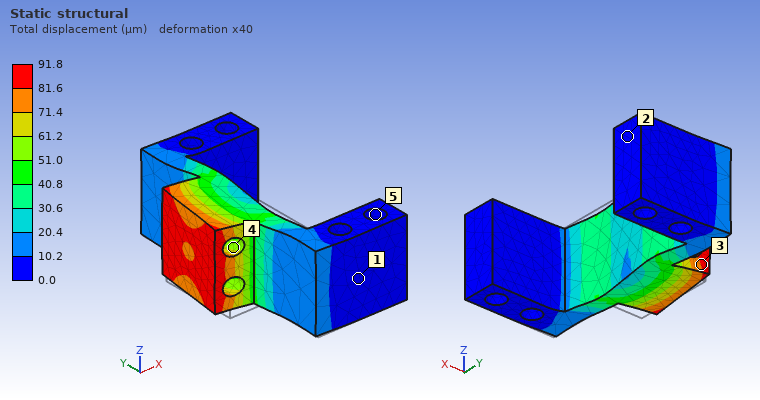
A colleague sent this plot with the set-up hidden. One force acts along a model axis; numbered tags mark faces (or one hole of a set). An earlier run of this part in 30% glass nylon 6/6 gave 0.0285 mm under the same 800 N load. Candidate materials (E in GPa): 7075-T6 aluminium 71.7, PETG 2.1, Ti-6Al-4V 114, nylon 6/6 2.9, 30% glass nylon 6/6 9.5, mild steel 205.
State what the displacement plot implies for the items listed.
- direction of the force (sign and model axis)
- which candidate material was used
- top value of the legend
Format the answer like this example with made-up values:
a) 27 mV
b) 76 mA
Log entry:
a) +Y
b) nylon 6/6
c) 91.8 µm
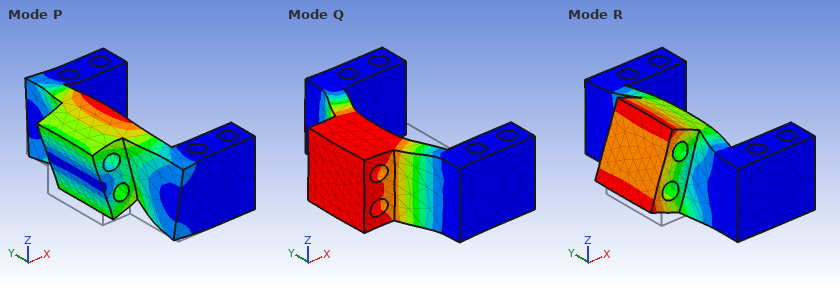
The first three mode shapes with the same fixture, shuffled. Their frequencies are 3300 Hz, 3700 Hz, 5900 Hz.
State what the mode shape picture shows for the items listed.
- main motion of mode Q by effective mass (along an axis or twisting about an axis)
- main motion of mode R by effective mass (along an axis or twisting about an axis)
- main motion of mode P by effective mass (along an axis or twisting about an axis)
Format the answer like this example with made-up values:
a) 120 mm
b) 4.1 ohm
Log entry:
a) along X
b) along Z
c) along Z
